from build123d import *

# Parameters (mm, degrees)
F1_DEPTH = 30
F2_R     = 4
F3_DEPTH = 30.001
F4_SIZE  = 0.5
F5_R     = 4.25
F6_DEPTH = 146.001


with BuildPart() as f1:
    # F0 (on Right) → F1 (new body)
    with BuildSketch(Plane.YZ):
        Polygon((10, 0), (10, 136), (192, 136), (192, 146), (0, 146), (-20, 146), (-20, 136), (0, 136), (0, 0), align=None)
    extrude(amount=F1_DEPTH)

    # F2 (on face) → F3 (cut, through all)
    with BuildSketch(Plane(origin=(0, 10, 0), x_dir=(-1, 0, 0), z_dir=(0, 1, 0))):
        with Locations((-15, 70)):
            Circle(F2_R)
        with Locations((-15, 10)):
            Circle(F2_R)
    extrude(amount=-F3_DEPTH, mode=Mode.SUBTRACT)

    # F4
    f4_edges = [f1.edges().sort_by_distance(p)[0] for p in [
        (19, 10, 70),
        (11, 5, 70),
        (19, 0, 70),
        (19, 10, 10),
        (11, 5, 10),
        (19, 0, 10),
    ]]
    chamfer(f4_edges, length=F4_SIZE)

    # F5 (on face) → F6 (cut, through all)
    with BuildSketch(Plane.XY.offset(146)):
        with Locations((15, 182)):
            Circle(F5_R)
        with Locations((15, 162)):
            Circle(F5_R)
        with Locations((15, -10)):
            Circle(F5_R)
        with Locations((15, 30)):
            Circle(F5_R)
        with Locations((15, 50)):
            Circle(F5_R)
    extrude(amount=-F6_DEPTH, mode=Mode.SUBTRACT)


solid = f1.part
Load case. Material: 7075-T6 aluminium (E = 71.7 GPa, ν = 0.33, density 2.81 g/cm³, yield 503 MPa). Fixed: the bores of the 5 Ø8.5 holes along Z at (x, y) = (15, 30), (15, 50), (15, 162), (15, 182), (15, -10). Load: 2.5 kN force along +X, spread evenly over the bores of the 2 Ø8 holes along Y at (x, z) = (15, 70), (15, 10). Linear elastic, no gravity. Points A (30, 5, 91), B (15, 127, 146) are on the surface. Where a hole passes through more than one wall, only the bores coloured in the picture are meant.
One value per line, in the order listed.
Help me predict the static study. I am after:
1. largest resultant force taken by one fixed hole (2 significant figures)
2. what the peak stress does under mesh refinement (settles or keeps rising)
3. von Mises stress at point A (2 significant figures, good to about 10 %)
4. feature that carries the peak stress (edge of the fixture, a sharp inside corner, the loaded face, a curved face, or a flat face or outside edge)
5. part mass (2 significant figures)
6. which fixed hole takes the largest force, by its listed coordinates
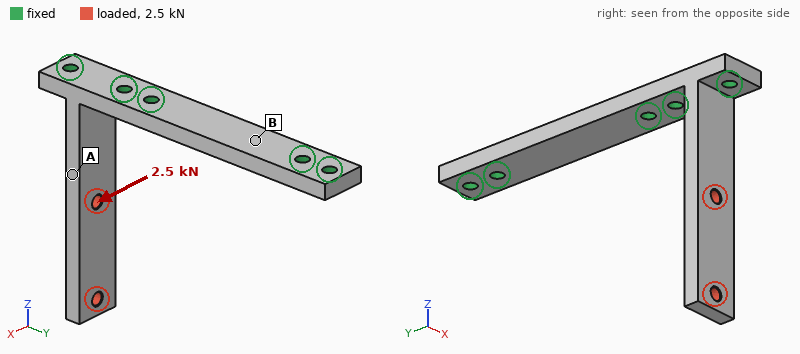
1.7 kN
keeps rising
85 MPa
edge of the fixture
280 g
(15, -10)
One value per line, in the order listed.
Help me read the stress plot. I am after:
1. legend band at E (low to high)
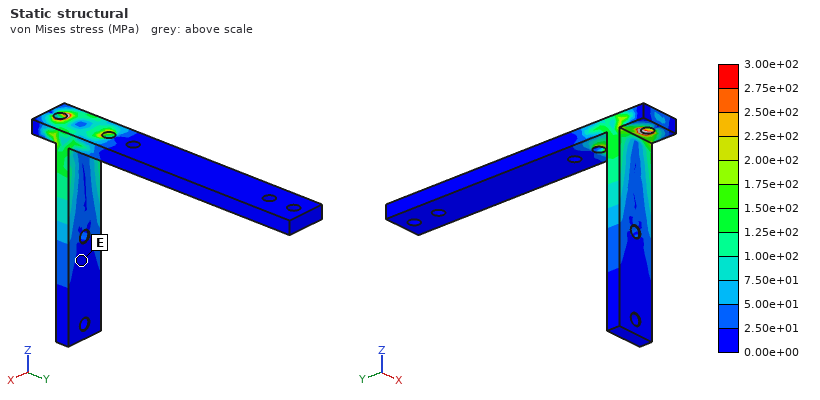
0.00e+00 to 2.50e+01 MPa
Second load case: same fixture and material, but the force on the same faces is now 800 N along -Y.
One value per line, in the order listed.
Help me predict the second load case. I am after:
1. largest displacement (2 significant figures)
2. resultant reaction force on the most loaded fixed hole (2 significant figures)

2.5 mm
2.8 kN
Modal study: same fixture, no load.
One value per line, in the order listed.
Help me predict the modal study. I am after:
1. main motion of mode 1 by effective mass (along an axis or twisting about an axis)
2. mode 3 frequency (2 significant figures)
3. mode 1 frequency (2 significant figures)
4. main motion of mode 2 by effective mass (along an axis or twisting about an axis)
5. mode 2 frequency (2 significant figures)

along Y
2500 Hz
420 Hz
along X
860 Hz
